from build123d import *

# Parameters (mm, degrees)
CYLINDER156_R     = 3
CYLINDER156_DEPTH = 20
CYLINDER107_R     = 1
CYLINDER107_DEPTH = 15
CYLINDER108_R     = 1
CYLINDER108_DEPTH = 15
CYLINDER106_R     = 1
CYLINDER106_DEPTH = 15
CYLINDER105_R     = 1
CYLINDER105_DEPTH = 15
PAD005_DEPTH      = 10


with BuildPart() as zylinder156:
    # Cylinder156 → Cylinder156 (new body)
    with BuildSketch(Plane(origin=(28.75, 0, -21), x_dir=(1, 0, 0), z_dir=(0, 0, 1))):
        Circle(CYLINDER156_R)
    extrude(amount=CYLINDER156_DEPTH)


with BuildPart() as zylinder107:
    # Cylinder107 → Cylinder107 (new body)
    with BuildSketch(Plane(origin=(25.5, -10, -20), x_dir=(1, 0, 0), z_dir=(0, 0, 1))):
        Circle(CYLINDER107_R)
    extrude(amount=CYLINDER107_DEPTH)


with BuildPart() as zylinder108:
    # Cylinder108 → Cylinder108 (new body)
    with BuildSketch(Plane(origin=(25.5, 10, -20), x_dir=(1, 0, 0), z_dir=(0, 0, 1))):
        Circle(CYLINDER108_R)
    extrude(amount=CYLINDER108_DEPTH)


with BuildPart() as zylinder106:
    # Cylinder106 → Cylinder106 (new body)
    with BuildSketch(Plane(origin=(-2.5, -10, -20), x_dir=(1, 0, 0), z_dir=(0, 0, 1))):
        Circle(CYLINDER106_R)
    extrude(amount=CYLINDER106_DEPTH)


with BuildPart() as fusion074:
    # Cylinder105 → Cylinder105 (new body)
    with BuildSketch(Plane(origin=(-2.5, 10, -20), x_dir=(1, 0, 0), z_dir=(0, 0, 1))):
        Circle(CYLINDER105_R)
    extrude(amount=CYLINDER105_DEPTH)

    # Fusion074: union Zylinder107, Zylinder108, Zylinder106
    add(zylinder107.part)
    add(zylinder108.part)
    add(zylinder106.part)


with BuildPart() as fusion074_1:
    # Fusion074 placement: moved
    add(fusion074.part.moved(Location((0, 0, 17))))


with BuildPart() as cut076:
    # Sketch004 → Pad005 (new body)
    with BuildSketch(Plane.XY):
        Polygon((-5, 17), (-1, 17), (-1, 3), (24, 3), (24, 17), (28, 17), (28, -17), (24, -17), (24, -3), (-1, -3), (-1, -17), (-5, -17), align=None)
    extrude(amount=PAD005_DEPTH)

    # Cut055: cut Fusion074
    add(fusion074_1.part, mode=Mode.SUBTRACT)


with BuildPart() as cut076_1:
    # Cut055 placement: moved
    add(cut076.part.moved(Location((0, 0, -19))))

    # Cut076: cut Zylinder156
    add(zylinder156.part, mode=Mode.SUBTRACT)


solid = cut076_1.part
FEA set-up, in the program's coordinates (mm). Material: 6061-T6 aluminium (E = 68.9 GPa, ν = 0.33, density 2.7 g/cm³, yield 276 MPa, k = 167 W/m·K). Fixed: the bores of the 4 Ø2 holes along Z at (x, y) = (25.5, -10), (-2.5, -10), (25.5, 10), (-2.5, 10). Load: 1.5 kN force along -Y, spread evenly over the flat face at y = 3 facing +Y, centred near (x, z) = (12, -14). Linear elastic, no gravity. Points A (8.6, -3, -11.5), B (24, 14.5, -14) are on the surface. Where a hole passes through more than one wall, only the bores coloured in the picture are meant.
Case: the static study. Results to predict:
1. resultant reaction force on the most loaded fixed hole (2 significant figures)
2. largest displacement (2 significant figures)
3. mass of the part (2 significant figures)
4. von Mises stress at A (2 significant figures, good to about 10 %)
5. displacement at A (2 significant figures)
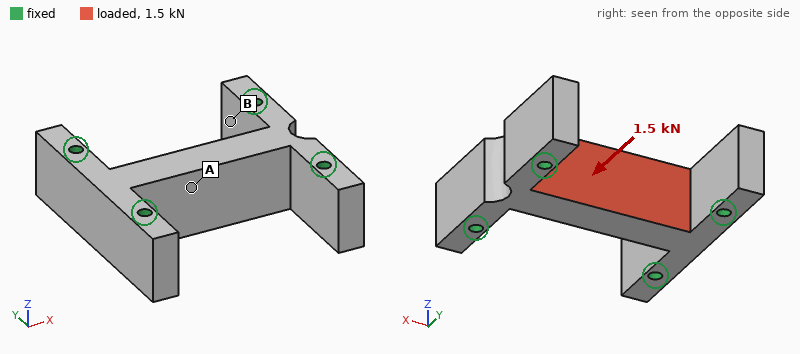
460 N
17 µm
11 g
37 MPa
15 µm
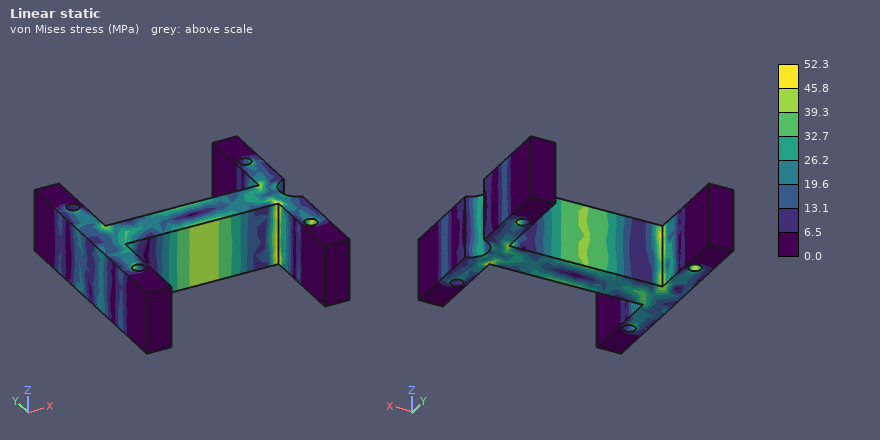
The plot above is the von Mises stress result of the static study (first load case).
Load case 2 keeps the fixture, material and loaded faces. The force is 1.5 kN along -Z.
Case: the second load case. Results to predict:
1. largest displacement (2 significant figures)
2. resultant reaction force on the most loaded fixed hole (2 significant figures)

25 µm
500 N
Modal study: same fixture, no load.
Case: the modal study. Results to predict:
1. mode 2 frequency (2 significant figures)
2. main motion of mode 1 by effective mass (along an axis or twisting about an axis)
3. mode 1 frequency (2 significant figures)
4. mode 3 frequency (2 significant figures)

25 kHz
along Z
24 kHz
26 kHz
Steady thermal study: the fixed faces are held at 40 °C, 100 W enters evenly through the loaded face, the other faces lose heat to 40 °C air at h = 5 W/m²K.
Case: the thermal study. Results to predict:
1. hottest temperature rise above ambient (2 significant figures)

69 K
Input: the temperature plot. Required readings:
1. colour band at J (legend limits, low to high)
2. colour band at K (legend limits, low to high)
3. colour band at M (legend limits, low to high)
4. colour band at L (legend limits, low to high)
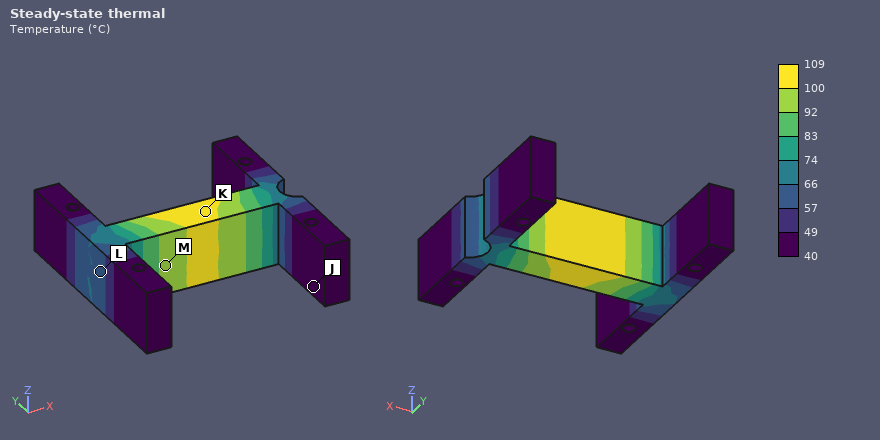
40 to 49 °C
100 to 109 °C
92 to 100 °C
57 to 66 °C
